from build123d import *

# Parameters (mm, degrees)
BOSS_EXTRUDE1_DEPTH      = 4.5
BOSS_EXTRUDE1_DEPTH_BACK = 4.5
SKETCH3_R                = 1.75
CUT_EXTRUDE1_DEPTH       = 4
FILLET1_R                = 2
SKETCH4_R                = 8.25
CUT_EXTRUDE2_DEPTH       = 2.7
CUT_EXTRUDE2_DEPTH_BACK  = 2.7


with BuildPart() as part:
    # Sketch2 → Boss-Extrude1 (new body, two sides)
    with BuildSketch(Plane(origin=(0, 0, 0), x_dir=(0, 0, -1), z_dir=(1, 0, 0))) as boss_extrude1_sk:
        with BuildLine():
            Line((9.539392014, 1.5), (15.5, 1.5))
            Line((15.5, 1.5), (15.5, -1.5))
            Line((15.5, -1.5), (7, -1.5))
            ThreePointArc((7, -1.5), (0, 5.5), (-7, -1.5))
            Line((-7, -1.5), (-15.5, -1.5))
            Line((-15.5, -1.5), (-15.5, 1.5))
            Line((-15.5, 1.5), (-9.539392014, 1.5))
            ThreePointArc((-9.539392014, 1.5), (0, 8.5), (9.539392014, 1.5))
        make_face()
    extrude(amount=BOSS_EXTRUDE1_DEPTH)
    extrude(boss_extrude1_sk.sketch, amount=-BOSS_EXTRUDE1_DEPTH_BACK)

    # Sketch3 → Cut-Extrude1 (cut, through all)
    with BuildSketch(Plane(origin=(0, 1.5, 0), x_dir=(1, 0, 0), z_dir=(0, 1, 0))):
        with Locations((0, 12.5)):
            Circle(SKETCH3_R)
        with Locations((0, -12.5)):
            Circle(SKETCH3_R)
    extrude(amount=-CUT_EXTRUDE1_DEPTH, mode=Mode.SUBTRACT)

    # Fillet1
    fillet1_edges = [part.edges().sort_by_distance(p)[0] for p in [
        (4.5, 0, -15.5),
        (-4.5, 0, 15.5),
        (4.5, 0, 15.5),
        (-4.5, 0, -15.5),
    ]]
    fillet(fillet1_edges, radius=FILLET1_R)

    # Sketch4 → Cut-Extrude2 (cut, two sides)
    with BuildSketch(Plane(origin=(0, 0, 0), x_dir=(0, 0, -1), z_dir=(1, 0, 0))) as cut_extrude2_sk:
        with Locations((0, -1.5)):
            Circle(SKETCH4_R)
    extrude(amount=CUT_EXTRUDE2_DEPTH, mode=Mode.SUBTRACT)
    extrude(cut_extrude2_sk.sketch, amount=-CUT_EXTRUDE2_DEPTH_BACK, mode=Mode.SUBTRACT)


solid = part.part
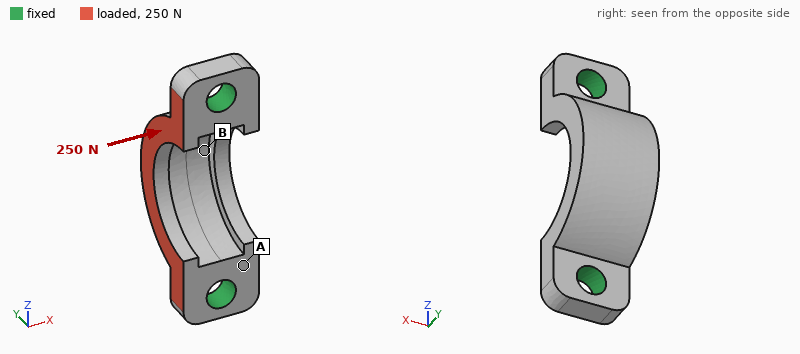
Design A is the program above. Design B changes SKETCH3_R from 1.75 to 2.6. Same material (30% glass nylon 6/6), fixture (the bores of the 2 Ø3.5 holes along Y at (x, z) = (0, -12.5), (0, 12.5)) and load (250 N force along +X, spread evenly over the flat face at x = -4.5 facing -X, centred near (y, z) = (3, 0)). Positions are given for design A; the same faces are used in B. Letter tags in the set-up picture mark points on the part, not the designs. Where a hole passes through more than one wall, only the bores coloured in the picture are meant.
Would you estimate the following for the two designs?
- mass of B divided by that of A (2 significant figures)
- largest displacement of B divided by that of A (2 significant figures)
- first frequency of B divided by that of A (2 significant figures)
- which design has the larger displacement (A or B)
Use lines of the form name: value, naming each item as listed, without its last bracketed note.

mass of B divided by that of A: 0.91
largest displacement of B divided by that of A: 0.64
first frequency of B divided by that of A: 1.2
which design has the larger displacement: A
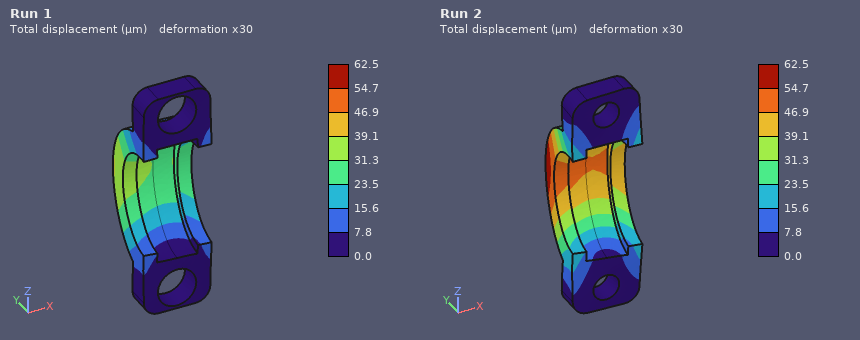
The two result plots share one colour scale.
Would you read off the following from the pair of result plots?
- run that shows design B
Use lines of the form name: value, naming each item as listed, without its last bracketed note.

run that shows design B: Run 1
